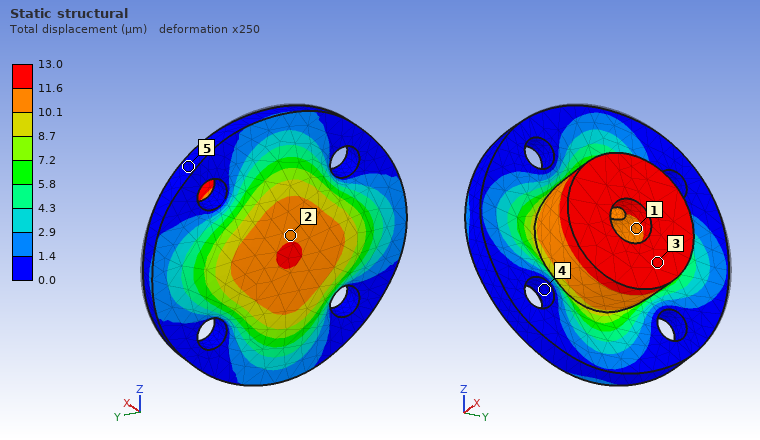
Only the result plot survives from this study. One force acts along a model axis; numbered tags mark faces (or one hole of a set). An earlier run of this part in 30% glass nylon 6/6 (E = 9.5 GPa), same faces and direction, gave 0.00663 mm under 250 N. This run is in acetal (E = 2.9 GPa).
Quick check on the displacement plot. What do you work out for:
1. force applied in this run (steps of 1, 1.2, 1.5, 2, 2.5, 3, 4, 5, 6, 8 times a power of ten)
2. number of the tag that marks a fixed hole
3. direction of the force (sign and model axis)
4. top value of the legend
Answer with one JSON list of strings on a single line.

["150 N", "4", "-X", "13.0 µm"]
